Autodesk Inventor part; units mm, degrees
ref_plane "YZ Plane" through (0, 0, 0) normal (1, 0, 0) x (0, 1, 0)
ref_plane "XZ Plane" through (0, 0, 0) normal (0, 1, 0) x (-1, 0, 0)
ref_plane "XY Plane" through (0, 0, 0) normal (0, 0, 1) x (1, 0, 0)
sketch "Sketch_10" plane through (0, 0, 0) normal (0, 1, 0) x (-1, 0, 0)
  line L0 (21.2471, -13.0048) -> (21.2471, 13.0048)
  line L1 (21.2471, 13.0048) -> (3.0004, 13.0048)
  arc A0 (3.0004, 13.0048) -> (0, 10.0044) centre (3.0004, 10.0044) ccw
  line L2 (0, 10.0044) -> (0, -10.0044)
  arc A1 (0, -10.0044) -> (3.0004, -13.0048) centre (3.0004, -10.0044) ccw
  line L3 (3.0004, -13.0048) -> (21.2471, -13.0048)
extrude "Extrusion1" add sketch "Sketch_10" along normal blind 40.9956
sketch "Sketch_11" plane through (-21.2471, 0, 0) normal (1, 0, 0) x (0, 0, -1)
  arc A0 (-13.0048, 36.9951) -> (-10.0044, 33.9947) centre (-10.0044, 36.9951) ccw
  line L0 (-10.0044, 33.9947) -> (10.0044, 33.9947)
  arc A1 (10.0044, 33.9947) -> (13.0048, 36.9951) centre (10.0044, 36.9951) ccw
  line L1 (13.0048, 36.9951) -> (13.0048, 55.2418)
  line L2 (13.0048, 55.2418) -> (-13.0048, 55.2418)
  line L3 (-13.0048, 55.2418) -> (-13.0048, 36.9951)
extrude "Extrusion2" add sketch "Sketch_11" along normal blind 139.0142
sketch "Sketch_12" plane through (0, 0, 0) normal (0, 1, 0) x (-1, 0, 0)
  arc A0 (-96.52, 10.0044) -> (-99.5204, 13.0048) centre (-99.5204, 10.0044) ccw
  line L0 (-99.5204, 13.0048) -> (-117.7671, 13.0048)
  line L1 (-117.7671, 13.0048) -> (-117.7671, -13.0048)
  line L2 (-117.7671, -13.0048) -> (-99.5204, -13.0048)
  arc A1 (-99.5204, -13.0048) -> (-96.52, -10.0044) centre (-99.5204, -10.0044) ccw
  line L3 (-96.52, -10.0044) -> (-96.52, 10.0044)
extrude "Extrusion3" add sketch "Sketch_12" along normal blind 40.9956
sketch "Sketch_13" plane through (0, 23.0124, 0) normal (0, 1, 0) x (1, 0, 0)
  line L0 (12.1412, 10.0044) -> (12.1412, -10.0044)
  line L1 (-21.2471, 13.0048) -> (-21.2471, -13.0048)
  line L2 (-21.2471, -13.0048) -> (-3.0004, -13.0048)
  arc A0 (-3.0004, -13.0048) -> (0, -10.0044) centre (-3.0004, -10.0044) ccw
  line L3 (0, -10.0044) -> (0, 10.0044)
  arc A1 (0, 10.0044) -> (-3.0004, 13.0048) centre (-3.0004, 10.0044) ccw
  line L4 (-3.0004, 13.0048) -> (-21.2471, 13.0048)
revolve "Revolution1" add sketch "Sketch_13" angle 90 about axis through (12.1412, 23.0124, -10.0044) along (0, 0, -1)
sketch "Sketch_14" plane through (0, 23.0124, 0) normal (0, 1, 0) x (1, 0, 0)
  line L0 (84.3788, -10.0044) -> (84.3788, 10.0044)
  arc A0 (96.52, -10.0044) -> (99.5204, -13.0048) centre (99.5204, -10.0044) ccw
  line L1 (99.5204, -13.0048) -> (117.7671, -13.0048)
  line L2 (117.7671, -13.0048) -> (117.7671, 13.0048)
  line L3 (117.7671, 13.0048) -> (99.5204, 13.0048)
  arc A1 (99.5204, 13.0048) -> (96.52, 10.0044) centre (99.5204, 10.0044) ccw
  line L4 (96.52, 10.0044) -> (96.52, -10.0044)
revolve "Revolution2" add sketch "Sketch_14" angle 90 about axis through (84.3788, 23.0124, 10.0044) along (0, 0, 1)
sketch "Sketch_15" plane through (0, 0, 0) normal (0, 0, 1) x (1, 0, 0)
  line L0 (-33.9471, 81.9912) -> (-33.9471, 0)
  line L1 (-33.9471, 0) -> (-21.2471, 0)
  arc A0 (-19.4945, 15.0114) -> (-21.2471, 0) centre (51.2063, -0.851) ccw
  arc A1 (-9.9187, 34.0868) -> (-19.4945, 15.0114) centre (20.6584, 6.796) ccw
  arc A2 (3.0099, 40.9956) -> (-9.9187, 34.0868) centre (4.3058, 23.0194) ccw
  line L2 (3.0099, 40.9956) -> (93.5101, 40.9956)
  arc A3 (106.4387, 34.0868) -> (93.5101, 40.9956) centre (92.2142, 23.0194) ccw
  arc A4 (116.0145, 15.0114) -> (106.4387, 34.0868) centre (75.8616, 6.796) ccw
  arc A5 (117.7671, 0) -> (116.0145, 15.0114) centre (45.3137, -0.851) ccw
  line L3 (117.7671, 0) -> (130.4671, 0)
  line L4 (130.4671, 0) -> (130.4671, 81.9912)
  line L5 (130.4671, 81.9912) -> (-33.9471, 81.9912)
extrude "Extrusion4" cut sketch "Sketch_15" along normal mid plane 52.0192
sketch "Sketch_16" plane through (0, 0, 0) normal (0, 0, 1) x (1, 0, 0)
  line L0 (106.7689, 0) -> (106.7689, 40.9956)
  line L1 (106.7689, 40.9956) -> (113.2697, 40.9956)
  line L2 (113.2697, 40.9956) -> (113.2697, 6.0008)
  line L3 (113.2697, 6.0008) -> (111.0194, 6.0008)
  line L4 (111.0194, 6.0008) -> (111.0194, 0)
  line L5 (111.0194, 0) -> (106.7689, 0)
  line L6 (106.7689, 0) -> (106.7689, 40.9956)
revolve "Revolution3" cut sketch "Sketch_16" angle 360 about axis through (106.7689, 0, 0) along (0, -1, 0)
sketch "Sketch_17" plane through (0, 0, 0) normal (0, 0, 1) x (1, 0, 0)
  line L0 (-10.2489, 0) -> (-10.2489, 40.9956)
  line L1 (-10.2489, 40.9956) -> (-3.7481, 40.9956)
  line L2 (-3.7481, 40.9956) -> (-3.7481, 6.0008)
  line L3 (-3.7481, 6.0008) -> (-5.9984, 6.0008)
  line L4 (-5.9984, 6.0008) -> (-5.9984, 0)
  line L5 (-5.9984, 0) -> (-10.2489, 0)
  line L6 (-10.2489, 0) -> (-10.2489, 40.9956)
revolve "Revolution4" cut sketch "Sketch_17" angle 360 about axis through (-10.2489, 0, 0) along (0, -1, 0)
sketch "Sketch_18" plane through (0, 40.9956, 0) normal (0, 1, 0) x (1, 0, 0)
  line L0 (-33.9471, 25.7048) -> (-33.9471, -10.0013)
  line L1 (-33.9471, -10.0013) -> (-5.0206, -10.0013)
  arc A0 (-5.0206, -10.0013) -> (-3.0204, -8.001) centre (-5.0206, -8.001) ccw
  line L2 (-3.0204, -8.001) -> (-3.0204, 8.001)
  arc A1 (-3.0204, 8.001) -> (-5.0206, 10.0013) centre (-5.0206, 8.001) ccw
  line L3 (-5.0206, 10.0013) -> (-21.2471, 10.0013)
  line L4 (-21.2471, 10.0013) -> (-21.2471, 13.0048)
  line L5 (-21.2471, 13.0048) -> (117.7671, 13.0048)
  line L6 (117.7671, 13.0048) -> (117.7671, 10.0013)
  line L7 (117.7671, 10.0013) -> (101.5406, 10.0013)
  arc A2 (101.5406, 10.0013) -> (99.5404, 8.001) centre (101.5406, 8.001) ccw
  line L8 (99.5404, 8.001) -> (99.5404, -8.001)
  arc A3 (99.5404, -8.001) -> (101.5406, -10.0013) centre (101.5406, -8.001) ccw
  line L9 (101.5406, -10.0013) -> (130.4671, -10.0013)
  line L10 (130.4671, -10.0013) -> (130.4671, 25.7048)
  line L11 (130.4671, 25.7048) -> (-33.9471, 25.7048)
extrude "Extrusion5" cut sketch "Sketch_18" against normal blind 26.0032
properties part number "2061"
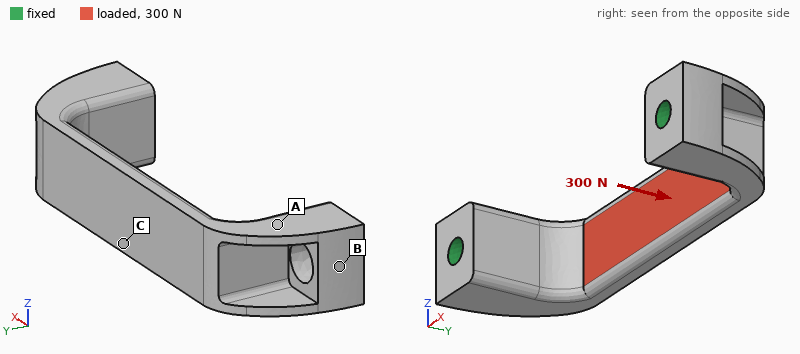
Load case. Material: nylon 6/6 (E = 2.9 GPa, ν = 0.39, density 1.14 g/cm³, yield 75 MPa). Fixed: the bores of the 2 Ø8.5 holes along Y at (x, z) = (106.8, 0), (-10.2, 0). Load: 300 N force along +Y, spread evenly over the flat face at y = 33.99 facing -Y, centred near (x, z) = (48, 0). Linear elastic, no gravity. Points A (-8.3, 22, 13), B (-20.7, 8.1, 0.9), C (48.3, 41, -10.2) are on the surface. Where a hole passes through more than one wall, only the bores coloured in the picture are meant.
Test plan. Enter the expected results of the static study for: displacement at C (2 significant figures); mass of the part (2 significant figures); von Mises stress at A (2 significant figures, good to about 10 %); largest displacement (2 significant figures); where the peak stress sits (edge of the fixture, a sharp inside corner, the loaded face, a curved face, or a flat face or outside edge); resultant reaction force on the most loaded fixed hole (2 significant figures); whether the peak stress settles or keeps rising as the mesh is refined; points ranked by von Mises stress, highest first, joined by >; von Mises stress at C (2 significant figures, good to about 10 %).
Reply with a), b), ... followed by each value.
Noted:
a) 0.52 mm
b) 44 g
c) 2.6 MPa
d) 0.53 mm
e) a sharp inside corner
f) 200 N
g) keeps rising
h) C > A > B
i) 8.2 MPa
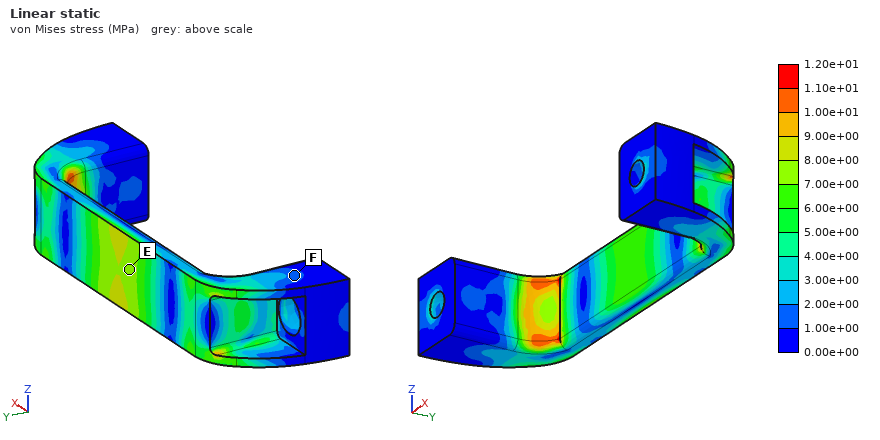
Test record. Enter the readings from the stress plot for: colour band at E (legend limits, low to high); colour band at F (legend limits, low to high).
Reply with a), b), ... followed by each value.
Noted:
a) 7.00e+00 to 8.00e+00 MPa
b) 1.00e+00 to 2.00e+00 MPa
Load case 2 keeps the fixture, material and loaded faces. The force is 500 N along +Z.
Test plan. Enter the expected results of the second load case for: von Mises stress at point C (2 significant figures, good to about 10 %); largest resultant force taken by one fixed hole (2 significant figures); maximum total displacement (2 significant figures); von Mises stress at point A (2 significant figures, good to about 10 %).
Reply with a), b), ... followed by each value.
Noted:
a) 6.4 MPa
b) 250 N
c) 0.62 mm
d) 4.1 MPa
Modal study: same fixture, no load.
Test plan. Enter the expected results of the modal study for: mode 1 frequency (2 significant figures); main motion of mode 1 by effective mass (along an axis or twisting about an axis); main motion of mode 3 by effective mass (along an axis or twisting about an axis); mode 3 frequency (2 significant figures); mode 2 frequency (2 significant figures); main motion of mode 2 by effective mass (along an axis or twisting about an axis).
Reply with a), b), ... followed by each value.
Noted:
a) 970 Hz
b) along Z
c) along X
d) 1100 Hz
e) 1100 Hz
f) along Y
